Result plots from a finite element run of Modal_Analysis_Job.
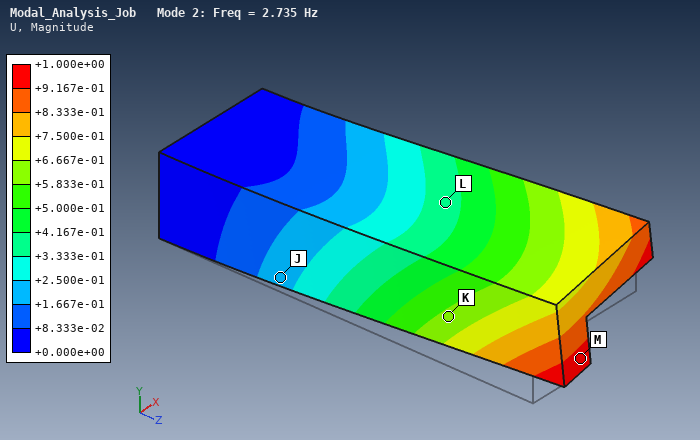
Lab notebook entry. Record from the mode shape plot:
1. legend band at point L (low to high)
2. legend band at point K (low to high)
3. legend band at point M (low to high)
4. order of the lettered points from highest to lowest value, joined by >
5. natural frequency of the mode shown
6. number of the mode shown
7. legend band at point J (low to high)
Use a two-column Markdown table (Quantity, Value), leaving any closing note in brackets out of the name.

| Quantity | Value |
|---|---|
| legend band at point L | +3.333e-01 to +4.167e-01 |
| legend band at point K | +5.833e-01 to +6.667e-01 |
| legend band at point M | +9.167e-01 to +1.000e+00 |
| order of the lettered points from highest to lowest value, joined by > | M > K > L > J |
| natural frequency of the mode shown | 2.735 Hz |
| number of the mode shown | 2 |
| legend band at point J | +1.667e-01 to +2.500e-01 |
